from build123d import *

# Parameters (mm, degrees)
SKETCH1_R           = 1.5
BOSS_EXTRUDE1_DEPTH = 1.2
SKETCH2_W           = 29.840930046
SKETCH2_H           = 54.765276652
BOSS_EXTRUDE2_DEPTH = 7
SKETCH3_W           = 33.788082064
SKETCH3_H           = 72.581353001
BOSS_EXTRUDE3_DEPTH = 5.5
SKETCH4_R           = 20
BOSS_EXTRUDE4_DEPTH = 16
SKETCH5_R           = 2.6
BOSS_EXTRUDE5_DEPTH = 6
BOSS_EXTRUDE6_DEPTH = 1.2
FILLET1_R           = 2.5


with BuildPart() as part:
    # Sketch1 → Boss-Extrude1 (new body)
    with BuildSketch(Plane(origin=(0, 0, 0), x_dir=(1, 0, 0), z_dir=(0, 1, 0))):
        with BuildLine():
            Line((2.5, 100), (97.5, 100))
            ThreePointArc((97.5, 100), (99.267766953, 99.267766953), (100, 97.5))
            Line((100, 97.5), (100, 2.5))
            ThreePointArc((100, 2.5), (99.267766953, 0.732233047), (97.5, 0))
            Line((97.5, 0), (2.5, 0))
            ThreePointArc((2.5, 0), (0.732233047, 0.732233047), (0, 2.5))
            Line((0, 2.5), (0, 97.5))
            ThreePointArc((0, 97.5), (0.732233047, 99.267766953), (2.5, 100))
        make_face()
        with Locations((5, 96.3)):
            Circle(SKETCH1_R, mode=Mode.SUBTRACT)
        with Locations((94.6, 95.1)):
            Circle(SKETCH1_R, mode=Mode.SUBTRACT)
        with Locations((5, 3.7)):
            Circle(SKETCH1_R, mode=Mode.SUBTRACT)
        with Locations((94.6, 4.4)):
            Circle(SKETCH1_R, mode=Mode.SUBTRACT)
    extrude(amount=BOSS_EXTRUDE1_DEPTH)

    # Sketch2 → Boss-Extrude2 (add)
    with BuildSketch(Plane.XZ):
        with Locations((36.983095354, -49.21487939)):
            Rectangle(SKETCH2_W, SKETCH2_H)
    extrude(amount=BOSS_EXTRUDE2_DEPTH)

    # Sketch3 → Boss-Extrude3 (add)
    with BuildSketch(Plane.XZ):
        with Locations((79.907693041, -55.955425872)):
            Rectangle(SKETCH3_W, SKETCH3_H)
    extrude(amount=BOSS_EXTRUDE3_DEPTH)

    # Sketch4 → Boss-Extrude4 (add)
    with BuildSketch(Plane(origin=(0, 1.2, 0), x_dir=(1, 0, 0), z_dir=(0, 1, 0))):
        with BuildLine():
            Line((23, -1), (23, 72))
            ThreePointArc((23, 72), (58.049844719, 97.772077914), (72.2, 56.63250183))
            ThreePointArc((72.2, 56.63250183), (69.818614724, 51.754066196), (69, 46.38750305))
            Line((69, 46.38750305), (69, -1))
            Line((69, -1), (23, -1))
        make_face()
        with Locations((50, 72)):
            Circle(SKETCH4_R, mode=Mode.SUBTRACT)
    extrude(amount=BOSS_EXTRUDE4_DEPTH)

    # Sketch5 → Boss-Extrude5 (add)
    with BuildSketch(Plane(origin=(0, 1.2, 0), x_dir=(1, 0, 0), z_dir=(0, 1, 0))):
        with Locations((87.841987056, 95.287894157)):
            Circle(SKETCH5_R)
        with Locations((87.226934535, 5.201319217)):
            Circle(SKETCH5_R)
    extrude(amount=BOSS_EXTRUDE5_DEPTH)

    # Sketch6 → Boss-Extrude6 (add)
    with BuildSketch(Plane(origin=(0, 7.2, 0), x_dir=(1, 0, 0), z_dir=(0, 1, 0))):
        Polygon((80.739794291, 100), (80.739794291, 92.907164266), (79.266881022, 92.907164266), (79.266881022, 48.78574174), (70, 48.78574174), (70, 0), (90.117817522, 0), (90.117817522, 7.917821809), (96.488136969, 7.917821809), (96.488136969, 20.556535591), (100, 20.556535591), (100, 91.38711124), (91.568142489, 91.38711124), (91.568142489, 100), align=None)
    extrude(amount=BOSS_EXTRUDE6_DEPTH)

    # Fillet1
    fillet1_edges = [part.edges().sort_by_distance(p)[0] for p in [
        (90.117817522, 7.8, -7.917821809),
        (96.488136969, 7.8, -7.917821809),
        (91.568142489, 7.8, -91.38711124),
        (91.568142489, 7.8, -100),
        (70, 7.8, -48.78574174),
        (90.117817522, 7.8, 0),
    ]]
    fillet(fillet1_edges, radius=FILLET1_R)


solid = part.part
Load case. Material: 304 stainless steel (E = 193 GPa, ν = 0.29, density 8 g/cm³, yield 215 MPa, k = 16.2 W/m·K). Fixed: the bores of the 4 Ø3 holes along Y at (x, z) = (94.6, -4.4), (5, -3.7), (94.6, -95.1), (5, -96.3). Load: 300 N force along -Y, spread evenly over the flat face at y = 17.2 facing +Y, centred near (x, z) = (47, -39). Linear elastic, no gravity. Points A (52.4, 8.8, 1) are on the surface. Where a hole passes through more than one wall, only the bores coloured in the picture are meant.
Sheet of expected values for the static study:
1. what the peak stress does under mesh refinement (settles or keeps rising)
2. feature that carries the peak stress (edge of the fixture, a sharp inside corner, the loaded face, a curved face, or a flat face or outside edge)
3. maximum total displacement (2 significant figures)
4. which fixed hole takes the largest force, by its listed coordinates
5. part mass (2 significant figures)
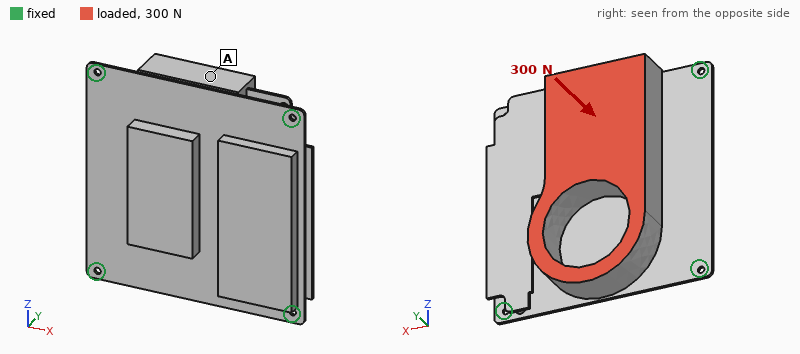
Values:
keeps rising
edge of the fixture
0.10 mm
(5, -3.7)
750 g
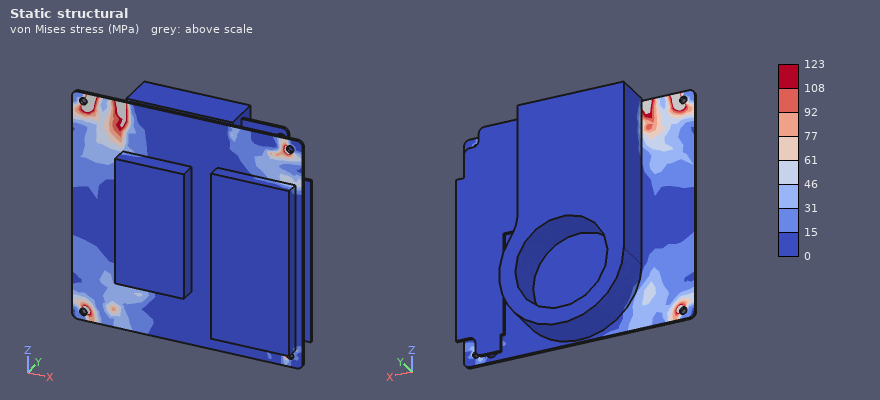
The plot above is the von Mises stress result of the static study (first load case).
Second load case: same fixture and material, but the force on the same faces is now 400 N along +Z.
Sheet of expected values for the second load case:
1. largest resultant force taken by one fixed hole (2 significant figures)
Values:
130 N
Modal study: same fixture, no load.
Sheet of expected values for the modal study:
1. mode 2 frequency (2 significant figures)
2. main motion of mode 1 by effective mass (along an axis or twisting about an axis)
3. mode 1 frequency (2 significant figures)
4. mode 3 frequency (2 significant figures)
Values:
670 Hz
along Y
410 Hz
760 Hz
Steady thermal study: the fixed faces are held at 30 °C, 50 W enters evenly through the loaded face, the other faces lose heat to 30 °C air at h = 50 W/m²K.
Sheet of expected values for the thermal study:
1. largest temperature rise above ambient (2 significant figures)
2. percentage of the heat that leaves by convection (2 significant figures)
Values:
76 K
96 %
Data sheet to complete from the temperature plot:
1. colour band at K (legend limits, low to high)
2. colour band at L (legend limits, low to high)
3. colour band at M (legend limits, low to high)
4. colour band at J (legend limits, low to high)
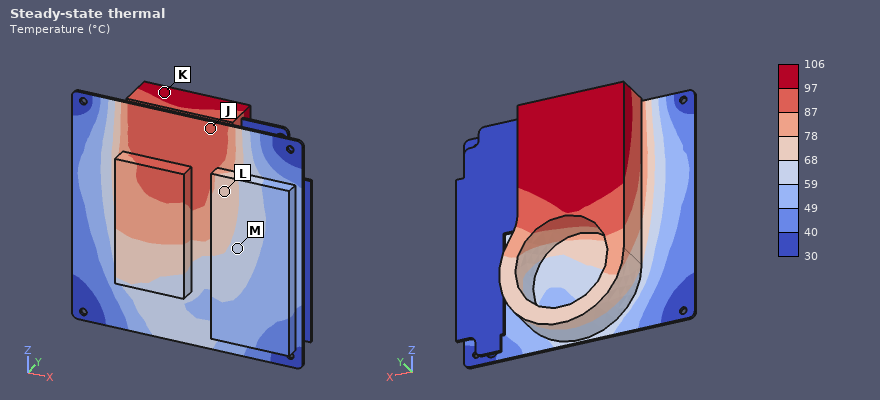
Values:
97 to 106 °C
68 to 78 °C
59 to 68 °C
87 to 97 °C
